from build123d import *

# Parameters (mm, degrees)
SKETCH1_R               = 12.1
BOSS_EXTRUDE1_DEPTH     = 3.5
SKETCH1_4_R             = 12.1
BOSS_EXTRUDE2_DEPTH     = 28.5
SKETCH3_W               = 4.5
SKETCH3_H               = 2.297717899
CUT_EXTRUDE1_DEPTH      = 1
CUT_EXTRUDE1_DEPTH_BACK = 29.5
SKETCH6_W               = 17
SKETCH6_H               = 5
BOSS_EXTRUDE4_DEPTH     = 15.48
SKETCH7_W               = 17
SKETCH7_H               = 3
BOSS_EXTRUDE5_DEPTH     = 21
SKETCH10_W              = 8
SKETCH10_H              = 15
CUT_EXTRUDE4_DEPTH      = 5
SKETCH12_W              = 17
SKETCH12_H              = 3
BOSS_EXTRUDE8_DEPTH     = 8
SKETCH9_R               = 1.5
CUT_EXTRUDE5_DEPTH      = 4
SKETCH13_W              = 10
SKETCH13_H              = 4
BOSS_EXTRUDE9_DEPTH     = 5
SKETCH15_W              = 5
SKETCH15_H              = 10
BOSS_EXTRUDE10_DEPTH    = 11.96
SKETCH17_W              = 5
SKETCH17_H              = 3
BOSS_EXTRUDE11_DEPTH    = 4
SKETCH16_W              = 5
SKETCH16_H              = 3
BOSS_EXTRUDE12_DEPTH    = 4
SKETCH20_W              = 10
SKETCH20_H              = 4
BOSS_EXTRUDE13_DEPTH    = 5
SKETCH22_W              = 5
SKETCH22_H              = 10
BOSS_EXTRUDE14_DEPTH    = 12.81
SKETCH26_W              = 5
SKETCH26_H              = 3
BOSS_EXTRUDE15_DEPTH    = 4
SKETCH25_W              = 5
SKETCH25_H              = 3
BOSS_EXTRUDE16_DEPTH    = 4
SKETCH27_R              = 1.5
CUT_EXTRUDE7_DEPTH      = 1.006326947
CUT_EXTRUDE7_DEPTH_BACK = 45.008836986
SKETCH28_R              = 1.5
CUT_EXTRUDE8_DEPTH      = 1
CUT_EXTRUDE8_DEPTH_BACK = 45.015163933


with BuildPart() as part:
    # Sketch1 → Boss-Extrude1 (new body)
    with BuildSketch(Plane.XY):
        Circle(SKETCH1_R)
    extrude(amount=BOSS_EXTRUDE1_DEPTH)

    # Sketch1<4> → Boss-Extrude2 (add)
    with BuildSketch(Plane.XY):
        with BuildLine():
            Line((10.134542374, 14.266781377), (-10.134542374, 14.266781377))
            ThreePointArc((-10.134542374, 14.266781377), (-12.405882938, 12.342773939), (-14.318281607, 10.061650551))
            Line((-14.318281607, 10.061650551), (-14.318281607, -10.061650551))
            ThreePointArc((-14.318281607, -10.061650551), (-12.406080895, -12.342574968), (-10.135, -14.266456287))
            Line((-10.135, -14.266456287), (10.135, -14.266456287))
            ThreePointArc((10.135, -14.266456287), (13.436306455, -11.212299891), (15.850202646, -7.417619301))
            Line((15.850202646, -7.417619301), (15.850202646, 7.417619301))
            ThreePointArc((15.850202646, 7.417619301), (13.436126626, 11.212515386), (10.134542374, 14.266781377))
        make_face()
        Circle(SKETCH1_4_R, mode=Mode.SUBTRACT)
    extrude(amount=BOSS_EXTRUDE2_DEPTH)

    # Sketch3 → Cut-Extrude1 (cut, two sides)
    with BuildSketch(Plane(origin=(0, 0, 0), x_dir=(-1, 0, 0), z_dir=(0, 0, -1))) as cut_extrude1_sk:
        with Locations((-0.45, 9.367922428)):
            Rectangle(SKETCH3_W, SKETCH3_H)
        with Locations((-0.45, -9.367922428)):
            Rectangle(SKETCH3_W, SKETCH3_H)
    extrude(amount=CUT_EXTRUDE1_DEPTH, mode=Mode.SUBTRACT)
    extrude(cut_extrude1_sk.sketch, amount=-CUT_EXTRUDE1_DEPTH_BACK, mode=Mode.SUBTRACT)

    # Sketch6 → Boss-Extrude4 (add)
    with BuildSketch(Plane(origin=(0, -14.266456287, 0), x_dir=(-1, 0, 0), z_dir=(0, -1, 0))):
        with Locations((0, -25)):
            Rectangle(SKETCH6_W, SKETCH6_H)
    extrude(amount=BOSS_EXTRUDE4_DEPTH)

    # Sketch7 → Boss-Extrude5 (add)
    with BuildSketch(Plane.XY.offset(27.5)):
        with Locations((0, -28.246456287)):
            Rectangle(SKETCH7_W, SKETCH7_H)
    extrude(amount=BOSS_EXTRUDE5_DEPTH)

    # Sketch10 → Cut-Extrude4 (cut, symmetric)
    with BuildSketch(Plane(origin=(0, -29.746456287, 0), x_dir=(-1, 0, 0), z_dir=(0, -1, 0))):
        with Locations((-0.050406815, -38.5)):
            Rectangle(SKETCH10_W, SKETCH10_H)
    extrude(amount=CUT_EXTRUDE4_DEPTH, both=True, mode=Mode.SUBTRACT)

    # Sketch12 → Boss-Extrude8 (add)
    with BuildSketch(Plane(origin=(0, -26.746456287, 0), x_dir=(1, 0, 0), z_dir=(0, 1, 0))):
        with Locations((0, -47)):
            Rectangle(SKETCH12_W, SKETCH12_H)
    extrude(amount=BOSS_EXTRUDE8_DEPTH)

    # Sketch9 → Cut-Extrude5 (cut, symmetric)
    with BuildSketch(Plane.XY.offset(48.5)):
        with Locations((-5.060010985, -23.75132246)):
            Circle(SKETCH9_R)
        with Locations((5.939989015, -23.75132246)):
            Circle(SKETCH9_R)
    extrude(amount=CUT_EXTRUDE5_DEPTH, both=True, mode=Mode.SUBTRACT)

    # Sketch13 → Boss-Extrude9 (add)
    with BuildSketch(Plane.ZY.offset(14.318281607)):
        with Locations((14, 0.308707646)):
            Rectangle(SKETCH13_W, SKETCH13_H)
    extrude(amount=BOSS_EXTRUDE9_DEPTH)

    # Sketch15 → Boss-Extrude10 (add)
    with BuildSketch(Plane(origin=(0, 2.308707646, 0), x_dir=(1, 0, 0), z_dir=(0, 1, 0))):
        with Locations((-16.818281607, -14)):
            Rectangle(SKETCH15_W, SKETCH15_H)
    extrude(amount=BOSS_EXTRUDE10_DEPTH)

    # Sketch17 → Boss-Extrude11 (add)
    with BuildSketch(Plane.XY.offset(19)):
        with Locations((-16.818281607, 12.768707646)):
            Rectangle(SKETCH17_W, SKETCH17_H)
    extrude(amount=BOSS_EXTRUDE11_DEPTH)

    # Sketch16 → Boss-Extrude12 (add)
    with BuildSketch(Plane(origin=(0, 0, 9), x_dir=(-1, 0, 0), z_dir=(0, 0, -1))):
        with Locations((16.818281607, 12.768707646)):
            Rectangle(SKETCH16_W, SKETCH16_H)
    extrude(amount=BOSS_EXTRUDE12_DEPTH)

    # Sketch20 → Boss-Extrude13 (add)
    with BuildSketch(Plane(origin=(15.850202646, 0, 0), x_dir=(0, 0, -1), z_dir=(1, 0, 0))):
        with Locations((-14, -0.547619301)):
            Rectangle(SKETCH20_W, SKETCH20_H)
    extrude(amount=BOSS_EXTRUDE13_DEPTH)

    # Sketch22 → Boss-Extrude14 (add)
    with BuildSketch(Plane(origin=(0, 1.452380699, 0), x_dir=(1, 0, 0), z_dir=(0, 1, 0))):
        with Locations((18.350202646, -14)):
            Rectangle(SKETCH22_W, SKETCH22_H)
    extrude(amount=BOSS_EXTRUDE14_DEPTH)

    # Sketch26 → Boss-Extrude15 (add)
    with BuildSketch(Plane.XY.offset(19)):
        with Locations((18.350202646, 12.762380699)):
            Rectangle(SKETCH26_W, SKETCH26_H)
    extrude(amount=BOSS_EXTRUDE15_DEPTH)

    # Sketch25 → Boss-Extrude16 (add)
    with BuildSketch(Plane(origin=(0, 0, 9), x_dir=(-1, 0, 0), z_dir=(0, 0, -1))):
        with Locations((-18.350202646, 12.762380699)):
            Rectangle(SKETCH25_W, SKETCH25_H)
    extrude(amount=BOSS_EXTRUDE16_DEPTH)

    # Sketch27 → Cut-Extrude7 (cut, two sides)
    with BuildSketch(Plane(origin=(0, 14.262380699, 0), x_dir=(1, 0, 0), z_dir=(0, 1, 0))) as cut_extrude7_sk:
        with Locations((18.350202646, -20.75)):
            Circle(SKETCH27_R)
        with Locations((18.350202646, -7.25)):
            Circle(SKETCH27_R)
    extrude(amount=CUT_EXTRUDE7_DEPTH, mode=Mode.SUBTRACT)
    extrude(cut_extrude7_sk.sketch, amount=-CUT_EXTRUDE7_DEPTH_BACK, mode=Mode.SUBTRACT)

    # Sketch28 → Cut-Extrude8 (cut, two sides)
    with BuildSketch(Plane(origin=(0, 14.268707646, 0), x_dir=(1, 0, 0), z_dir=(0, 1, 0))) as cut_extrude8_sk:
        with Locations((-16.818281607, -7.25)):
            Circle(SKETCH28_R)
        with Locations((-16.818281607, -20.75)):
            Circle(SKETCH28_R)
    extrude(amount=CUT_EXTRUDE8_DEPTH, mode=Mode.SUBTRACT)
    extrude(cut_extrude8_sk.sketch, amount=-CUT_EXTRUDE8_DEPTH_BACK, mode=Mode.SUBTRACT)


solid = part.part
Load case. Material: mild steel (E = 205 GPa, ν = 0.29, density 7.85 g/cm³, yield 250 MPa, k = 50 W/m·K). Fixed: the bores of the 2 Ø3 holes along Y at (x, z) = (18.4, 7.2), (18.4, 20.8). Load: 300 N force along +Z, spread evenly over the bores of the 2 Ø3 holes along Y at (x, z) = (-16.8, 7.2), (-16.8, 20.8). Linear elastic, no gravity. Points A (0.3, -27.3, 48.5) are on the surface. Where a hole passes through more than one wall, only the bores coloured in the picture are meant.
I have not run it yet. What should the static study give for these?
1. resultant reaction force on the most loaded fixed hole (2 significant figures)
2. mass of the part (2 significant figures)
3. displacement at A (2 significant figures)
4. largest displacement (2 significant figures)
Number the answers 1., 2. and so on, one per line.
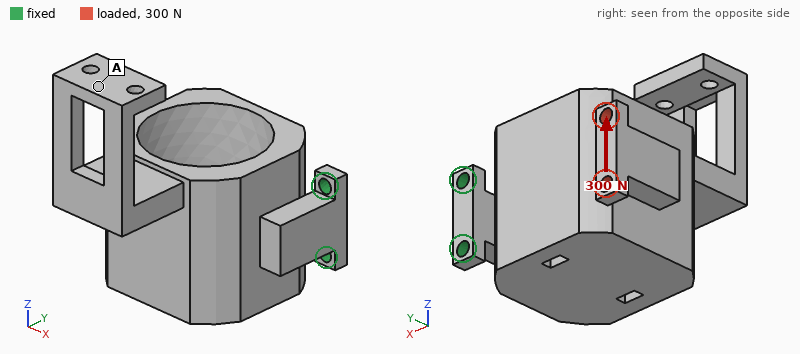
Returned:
1. 950 N
2. 120 g
3. 0.11 mm
4. 0.13 mm
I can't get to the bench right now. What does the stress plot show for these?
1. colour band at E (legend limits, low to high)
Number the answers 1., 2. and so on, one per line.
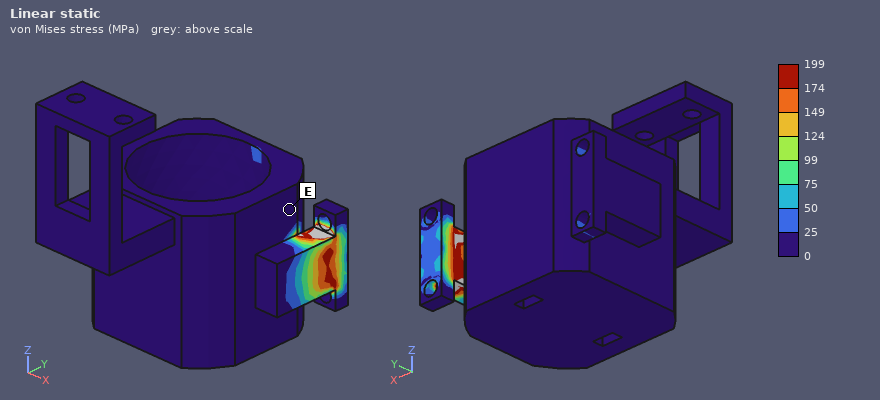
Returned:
1. 0 to 25 MPa
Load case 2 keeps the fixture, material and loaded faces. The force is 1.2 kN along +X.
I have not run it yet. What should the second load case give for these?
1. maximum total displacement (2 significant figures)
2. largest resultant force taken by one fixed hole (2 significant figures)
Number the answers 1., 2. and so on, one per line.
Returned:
1. 94 µm
2. 600 N
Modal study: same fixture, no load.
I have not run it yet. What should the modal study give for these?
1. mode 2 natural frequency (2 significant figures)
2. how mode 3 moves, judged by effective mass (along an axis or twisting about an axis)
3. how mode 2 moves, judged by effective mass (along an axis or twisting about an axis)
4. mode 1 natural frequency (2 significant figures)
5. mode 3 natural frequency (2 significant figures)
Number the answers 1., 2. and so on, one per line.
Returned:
1. 1100 Hz
2. twisting about X
3. along Z
4. 620 Hz
5. 1900 Hz
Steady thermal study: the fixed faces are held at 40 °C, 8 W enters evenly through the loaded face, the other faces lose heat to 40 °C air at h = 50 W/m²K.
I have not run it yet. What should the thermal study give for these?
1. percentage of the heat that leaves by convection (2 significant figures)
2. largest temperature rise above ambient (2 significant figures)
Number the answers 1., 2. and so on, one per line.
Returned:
1. 76 %
2. 67 K
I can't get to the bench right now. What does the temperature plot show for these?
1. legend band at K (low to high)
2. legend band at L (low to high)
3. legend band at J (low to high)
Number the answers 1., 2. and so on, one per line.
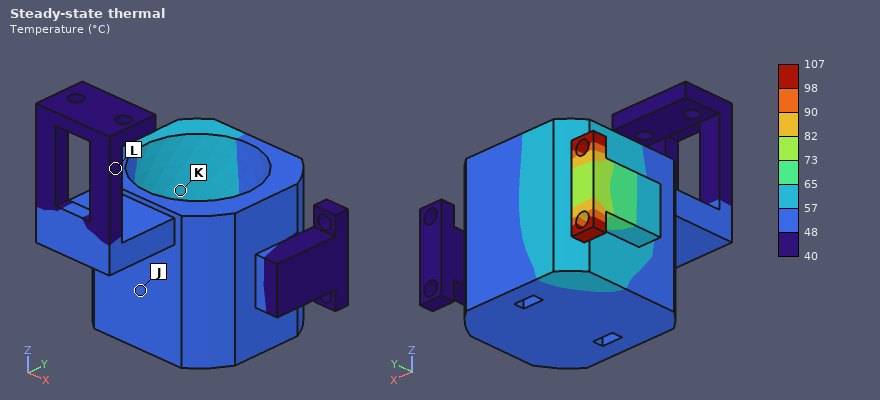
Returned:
1. 57 to 65 °C
2. 40 to 48 °C
3. 48 to 57 °C
